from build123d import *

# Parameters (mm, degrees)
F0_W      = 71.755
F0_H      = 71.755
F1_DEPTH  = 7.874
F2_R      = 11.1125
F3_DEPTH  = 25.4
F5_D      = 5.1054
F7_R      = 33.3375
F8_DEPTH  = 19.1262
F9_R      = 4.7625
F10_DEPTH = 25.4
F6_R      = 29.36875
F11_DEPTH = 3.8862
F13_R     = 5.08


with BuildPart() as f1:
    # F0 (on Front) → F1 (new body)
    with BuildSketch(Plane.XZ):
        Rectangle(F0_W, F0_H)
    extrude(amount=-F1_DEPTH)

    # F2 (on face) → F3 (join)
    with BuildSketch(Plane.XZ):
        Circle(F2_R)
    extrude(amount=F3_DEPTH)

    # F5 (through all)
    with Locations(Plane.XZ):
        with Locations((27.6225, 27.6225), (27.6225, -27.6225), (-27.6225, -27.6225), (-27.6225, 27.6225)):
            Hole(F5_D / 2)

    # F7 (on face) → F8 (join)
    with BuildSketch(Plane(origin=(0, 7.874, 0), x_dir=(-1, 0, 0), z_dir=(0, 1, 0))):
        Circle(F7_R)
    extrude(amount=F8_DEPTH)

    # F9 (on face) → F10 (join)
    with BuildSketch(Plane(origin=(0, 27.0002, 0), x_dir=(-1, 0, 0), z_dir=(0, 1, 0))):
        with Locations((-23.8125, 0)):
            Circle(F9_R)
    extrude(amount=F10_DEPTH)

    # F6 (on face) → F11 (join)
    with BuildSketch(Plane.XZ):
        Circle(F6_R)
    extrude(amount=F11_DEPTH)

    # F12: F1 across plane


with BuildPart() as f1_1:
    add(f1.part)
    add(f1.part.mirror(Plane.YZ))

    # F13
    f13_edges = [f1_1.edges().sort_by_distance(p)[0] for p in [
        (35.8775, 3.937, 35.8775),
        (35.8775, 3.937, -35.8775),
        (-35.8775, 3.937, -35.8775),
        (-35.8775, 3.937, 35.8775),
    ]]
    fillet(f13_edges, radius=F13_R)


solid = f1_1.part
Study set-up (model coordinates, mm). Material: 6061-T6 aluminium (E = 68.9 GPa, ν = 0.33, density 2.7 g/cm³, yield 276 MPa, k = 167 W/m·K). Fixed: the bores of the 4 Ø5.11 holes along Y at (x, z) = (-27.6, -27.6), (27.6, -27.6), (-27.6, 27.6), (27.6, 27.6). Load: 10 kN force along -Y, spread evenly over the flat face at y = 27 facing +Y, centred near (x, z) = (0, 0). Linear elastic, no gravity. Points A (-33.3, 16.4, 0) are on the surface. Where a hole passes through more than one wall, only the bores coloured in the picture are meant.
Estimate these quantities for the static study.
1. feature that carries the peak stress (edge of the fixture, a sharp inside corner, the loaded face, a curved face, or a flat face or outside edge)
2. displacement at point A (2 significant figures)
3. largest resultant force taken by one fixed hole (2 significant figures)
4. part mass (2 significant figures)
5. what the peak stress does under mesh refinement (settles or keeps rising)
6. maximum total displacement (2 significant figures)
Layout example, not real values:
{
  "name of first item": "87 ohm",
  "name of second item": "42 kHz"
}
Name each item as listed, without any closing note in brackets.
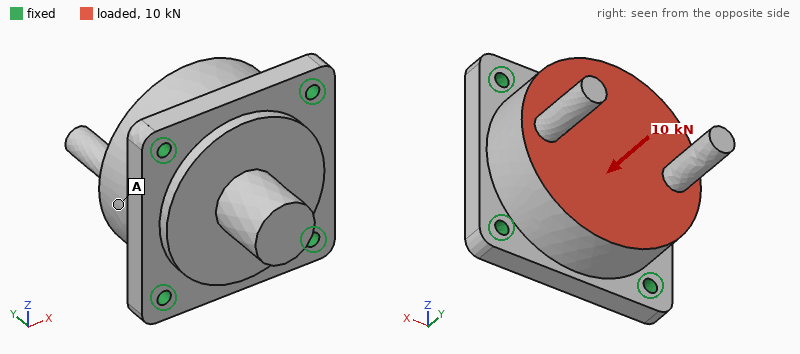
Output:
{
  "feature that carries the peak stress": "edge of the fixture",
  "displacement at point A": "10 µm",
  "largest resultant force taken by one fixed hole": "2.6 kN",
  "part mass": "350 g",
  "what the peak stress does under mesh refinement": "keeps rising",
  "maximum total displacement": "12 µm"
}
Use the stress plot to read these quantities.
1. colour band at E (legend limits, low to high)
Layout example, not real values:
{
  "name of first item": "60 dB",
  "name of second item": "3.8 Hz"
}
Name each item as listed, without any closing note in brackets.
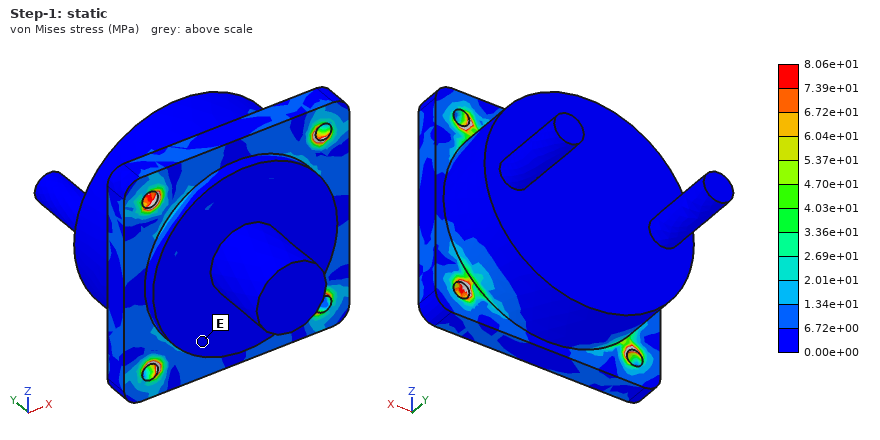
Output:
{
  "colour band at E": "0.00e+00 to 6.72e+00 MPa"
}
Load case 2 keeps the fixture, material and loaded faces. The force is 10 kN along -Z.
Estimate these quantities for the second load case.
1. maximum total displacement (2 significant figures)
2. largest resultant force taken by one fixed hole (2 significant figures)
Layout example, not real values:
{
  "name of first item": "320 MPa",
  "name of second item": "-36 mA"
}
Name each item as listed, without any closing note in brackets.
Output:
{
  "maximum total displacement": "20 µm",
  "largest resultant force taken by one fixed hole": "3.5 kN"
}
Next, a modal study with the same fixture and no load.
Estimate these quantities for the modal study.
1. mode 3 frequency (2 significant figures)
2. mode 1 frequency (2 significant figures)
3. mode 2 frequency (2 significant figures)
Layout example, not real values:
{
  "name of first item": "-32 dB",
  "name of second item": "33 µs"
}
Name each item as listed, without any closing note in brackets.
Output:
{
  "mode 3 frequency": "8300 Hz",
  "mode 1 frequency": "7800 Hz",
  "mode 2 frequency": "8000 Hz"
}
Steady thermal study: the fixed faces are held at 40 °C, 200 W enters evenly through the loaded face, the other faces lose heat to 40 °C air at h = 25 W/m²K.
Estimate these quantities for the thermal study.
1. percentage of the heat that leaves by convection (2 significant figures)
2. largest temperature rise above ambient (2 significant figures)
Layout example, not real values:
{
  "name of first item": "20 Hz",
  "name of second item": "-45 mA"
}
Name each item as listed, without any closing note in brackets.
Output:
{
  "percentage of the heat that leaves by convection": "3.4 %",
  "largest temperature rise above ambient": "26 K"
}
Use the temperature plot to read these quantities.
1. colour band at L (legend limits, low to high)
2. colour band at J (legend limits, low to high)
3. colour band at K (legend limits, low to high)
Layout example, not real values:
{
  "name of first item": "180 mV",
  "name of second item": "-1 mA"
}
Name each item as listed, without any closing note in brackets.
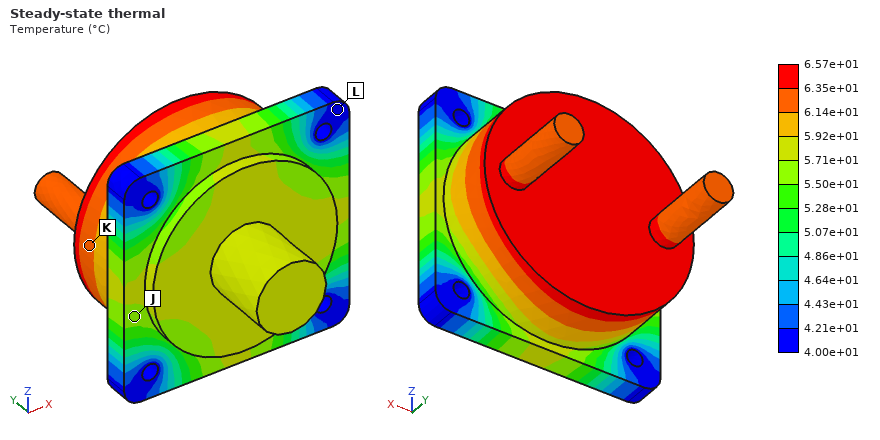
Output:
{
  "colour band at L": "4.00e+01 to 4.21e+01 °C",
  "colour band at J": "5.50e+01 to 5.71e+01 °C",
  "colour band at K": "6.14e+01 to 6.35e+01 °C"
}
